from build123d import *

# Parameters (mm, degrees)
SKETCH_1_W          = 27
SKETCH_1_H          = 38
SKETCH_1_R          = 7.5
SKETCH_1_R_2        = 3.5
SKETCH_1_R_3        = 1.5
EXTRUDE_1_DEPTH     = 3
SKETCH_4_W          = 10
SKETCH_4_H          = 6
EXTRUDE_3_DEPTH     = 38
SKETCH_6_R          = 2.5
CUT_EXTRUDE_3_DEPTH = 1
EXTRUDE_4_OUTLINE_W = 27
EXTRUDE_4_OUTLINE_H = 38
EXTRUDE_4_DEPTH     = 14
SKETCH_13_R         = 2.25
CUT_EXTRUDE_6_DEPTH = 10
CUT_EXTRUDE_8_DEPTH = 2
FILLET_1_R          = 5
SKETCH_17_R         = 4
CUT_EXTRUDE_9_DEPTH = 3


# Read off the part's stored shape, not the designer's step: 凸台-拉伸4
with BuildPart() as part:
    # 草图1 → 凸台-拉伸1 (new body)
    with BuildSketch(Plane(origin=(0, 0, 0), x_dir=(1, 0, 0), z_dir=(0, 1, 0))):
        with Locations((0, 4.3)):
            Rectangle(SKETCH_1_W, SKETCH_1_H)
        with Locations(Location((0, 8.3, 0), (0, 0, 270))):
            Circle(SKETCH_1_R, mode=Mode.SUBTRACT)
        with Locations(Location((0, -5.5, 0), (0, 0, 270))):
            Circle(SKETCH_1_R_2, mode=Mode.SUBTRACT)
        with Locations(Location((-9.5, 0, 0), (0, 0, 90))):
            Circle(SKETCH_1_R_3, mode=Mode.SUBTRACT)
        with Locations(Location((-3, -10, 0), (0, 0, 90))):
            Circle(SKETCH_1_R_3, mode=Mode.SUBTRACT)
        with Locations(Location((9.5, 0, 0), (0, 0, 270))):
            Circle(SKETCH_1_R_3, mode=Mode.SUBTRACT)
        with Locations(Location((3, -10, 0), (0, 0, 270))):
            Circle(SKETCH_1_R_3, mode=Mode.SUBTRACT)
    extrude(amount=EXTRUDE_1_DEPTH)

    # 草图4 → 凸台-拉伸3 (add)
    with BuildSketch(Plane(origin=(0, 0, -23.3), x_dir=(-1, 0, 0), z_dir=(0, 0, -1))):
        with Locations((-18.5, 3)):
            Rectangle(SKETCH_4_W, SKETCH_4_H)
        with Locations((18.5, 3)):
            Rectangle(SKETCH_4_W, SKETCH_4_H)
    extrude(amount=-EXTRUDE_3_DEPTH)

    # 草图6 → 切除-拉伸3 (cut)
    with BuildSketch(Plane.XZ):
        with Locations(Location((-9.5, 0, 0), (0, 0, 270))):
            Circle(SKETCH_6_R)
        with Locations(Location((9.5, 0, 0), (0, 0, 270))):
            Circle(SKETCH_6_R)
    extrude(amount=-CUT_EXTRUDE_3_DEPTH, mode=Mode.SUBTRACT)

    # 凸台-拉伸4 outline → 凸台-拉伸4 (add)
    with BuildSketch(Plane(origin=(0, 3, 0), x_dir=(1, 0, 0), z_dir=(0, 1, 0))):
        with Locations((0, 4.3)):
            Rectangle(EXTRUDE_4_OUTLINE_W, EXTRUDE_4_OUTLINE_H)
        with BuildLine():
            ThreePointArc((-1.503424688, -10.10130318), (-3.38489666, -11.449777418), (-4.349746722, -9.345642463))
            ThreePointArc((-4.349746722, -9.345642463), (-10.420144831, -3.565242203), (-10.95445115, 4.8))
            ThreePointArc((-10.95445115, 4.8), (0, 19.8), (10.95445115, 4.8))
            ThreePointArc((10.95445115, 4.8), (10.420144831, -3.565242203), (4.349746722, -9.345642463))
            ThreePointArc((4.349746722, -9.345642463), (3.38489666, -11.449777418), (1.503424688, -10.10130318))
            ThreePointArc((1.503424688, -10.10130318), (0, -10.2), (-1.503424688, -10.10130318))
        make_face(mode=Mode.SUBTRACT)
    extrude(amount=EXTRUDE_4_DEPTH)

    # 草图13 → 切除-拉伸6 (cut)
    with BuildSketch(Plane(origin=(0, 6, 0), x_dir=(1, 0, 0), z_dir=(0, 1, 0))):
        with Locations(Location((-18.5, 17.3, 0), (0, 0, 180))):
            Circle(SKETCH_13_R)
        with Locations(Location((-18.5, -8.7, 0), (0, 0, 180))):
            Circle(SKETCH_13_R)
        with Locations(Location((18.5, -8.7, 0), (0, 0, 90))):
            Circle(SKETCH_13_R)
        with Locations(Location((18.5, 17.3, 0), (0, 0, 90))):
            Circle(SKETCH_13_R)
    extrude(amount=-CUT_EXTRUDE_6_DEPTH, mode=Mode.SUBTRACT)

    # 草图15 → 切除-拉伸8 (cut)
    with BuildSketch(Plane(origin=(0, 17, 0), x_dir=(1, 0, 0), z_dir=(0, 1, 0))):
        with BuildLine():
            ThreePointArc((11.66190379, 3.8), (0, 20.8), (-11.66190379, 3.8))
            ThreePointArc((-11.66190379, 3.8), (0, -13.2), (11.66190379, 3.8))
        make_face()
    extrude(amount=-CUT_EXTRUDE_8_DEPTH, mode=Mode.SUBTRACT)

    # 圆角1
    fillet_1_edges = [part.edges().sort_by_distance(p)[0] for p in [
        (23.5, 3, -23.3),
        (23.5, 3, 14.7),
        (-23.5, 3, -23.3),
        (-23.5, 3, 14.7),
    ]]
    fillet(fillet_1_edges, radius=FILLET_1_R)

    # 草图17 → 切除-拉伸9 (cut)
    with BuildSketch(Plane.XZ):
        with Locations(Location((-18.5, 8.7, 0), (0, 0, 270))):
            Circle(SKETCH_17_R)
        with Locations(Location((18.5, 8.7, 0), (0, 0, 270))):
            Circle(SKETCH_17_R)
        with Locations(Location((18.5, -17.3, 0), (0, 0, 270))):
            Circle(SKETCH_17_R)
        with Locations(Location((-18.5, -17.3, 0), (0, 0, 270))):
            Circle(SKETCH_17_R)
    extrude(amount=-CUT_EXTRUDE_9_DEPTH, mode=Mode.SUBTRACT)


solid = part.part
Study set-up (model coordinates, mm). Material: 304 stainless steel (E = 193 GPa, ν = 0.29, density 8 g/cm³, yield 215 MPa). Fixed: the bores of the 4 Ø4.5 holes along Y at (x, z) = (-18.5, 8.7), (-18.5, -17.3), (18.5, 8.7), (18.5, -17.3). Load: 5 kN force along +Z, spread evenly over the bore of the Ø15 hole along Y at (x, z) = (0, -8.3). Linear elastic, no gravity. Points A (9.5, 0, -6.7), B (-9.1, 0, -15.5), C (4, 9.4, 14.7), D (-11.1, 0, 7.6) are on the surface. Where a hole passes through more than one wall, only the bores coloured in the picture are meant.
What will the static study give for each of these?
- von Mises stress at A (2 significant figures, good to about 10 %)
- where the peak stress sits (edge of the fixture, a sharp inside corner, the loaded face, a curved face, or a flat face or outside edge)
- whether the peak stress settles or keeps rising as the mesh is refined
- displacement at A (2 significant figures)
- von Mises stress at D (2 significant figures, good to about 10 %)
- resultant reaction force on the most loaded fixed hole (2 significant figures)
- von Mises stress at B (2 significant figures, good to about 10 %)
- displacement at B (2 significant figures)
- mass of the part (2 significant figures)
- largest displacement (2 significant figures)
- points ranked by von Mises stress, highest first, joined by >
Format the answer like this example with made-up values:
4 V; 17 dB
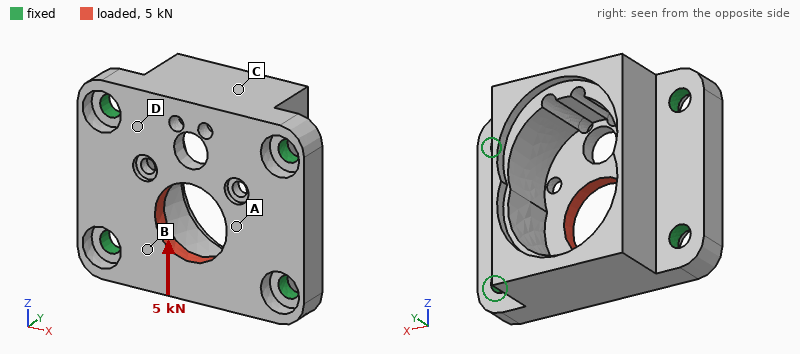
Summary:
51 MPa; edge of the fixture; keeps rising; 3.1 µm; 28 MPa; 1.4 kN; 40 MPa; 3.7 µm; 95 g; 7.4 µm; A > B > D > C
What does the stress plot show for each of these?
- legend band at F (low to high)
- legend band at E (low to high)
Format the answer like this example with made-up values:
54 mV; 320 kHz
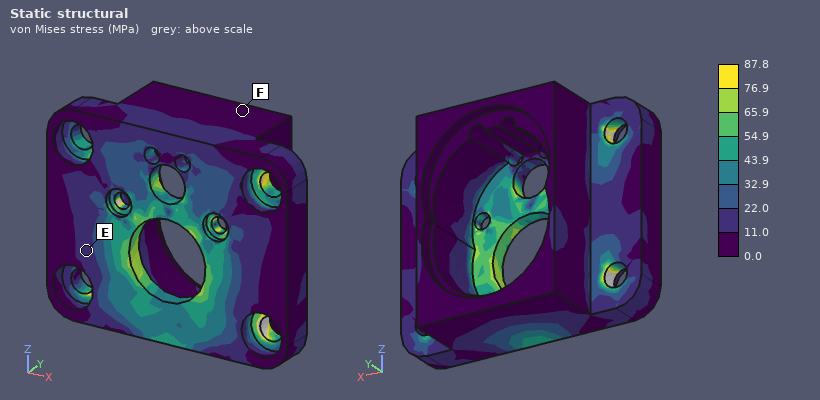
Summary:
0.0 to 11.0 MPa; 11.0 to 22.0 MPa
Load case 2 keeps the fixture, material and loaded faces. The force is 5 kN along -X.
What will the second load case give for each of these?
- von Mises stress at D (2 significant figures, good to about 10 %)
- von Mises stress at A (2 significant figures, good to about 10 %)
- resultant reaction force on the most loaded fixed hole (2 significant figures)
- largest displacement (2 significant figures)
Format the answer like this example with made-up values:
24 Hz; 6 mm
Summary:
24 MPa; 31 MPa; 1.6 kN; 4.8 µm
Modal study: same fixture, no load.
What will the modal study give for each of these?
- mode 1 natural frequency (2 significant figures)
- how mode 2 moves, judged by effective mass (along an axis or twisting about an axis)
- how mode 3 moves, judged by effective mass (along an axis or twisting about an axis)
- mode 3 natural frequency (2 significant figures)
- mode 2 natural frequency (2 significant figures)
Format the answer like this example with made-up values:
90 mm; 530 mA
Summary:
16 kHz; along Y; along Y; 22 kHz; 16 kHz
